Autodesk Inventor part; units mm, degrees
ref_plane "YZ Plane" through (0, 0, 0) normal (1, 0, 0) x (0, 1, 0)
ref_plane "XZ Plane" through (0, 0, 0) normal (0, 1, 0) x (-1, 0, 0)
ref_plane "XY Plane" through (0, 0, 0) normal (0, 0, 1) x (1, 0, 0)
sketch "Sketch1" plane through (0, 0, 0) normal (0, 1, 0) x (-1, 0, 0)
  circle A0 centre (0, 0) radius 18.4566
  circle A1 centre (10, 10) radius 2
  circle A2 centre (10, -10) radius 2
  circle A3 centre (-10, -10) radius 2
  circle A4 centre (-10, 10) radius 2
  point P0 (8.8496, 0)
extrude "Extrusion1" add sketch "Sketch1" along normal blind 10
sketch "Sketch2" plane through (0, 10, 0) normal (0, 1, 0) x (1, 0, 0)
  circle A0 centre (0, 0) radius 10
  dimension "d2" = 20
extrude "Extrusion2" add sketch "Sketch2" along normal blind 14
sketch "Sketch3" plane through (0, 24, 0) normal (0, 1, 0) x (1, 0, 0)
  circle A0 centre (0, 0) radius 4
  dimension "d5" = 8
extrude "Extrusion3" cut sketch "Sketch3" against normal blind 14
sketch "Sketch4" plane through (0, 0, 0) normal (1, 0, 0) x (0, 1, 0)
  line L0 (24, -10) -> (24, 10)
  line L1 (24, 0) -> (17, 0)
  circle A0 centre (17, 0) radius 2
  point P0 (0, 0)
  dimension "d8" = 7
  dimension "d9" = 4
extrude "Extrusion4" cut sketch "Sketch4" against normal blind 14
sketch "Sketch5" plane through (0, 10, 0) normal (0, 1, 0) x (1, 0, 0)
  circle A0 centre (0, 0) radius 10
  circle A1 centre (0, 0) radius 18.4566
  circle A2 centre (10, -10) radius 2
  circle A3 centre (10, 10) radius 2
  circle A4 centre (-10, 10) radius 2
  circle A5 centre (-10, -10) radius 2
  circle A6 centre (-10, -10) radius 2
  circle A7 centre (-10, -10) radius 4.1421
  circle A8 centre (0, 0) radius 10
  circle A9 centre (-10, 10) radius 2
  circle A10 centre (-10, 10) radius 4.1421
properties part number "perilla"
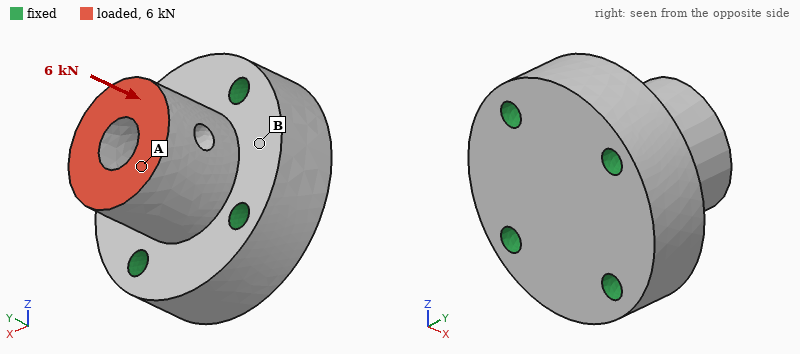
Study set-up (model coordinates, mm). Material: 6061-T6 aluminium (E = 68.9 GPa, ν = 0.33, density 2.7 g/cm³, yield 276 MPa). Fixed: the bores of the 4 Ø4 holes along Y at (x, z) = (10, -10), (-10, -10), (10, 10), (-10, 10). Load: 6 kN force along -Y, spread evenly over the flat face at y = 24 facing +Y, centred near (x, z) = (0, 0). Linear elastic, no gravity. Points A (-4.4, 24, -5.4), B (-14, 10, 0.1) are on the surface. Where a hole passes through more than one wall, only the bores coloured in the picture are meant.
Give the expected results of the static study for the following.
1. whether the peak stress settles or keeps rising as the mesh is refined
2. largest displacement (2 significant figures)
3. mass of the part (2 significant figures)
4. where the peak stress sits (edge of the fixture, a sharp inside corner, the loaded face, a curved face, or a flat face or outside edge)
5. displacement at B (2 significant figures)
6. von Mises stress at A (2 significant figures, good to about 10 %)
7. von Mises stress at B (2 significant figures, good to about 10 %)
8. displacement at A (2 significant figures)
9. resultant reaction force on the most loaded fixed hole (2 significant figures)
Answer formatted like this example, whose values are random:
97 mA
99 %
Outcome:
keeps rising
10 µm
37 g
edge of the fixture
1.6 µm
25 MPa
7.3 MPa
8.5 µm
1.6 kN
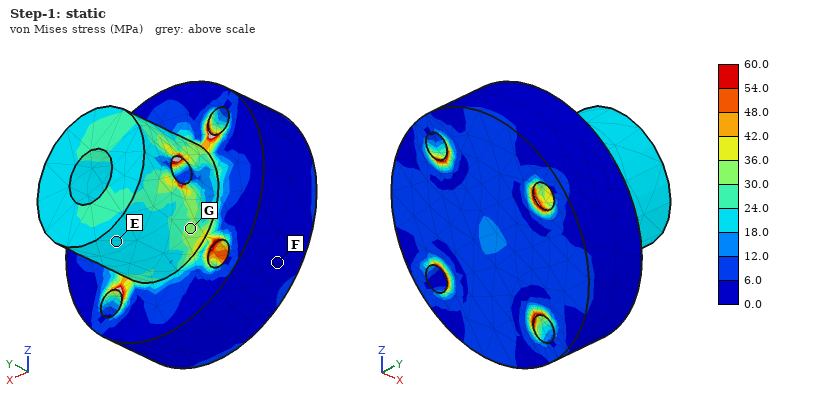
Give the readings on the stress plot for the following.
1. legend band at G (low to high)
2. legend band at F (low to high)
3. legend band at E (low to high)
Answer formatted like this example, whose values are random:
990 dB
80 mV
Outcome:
30.0 to 36.0 MPa
0.0 to 6.0 MPa
18.0 to 24.0 MPa
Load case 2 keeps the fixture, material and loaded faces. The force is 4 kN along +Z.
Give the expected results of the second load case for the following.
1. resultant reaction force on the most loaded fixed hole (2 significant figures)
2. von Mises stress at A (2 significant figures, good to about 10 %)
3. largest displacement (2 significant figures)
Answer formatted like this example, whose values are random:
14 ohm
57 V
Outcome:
2.1 kN
41 MPa
37 µm
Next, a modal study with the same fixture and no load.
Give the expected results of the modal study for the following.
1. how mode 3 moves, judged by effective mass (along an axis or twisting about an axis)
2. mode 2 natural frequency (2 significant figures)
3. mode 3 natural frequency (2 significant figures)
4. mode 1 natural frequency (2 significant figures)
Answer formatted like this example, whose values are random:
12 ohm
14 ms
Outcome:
along Y
29 kHz
43 kHz
28 kHz
